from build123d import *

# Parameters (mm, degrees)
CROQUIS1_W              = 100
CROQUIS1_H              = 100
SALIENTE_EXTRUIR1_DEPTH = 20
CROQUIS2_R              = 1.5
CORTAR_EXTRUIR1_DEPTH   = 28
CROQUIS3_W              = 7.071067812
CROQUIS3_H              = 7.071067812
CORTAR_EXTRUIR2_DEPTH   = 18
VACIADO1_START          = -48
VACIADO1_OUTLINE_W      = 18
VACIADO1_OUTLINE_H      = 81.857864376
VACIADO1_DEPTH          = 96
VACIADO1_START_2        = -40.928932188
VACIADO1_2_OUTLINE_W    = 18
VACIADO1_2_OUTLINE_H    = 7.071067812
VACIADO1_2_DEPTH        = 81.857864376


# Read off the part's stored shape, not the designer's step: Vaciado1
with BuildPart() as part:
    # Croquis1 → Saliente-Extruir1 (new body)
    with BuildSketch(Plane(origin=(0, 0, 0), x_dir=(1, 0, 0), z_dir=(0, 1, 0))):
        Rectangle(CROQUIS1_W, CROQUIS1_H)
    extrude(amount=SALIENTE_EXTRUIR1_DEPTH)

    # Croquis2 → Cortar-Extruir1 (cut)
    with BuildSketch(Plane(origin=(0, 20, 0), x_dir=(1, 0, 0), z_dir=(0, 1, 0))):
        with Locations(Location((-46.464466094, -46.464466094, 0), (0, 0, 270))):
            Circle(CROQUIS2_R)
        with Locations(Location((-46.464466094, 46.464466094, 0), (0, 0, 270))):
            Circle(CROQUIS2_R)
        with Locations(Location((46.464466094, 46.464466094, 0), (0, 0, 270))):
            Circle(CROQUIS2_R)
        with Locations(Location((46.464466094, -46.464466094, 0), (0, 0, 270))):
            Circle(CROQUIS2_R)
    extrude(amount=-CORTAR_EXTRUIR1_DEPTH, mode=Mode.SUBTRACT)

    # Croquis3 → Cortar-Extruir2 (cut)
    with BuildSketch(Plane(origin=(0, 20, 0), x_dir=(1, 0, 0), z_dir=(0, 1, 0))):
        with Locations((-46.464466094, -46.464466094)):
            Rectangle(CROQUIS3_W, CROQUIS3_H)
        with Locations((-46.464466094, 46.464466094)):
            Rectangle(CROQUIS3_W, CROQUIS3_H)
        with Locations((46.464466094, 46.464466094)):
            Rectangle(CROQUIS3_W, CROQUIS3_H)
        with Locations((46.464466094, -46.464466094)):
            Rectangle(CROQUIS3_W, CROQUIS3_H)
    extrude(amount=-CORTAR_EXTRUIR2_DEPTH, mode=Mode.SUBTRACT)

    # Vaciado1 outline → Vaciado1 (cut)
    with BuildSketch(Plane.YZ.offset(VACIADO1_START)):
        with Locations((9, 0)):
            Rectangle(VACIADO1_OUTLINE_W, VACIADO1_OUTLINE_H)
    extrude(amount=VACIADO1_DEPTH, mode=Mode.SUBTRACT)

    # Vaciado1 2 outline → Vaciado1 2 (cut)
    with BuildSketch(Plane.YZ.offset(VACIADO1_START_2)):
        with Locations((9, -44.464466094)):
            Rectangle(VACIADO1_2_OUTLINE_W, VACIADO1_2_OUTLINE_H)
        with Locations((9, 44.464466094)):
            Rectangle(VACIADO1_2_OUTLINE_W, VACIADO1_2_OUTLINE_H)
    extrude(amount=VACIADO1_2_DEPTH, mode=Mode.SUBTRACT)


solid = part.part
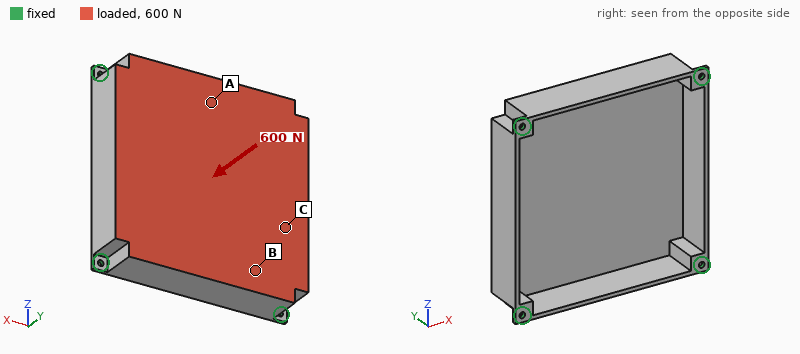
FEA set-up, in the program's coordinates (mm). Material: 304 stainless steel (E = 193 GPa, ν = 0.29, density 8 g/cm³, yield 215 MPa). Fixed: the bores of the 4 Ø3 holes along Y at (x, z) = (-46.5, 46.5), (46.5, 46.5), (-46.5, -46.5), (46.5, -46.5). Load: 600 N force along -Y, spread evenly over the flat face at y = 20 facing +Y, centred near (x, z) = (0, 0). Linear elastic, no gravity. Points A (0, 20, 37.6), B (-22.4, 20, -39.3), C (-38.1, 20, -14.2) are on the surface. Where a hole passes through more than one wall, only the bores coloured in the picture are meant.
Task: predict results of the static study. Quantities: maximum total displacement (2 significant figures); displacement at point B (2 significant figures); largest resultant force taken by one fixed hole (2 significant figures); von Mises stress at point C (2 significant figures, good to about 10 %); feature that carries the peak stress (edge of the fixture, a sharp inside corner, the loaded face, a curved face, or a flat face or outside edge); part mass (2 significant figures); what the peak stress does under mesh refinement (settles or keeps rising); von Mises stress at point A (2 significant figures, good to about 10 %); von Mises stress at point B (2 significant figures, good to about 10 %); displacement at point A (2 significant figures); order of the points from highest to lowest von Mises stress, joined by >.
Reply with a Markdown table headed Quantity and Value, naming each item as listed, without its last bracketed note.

| Quantity | Value |
|---|---|
| maximum total displacement | 92 µm |
| displacement at point B | 18 µm |
| largest resultant force taken by one fixed hole | 190 N |
| von Mises stress at point C | 13 MPa |
| feature that carries the peak stress | edge of the fixture |
| part mass | 270 g |
| what the peak stress does under mesh refinement | keeps rising |
| von Mises stress at point A | 9.0 MPa |
| von Mises stress at point B | 17 MPa |
| displacement at point A | 31 µm |
| order of the points from highest to lowest von Mises stress, joined by > | B > C > A |
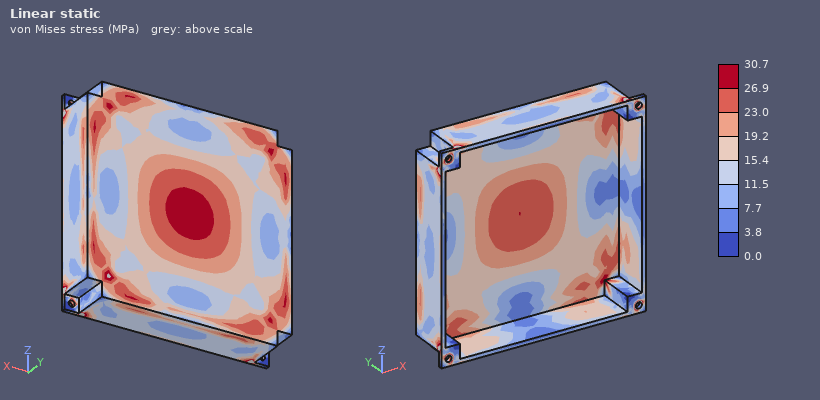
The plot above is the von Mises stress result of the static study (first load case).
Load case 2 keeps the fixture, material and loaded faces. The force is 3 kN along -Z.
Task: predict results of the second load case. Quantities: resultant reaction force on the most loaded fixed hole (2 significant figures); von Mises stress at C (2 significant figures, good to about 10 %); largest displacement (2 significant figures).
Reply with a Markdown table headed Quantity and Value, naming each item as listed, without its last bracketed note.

| Quantity | Value |
|---|---|
| resultant reaction force on the most loaded fixed hole | 810 N |
| von Mises stress at C | 12 MPa |
| largest displacement | 13 µm |
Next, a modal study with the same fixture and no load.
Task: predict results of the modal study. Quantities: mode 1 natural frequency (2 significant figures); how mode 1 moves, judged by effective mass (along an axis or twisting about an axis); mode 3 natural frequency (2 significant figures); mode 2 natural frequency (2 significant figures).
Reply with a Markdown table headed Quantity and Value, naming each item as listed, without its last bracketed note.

| Quantity | Value |
|---|---|
| mode 1 natural frequency | 1300 Hz |
| how mode 1 moves, judged by effective mass | along Y |
| mode 3 natural frequency | 2600 Hz |
| mode 2 natural frequency | 2600 Hz |
